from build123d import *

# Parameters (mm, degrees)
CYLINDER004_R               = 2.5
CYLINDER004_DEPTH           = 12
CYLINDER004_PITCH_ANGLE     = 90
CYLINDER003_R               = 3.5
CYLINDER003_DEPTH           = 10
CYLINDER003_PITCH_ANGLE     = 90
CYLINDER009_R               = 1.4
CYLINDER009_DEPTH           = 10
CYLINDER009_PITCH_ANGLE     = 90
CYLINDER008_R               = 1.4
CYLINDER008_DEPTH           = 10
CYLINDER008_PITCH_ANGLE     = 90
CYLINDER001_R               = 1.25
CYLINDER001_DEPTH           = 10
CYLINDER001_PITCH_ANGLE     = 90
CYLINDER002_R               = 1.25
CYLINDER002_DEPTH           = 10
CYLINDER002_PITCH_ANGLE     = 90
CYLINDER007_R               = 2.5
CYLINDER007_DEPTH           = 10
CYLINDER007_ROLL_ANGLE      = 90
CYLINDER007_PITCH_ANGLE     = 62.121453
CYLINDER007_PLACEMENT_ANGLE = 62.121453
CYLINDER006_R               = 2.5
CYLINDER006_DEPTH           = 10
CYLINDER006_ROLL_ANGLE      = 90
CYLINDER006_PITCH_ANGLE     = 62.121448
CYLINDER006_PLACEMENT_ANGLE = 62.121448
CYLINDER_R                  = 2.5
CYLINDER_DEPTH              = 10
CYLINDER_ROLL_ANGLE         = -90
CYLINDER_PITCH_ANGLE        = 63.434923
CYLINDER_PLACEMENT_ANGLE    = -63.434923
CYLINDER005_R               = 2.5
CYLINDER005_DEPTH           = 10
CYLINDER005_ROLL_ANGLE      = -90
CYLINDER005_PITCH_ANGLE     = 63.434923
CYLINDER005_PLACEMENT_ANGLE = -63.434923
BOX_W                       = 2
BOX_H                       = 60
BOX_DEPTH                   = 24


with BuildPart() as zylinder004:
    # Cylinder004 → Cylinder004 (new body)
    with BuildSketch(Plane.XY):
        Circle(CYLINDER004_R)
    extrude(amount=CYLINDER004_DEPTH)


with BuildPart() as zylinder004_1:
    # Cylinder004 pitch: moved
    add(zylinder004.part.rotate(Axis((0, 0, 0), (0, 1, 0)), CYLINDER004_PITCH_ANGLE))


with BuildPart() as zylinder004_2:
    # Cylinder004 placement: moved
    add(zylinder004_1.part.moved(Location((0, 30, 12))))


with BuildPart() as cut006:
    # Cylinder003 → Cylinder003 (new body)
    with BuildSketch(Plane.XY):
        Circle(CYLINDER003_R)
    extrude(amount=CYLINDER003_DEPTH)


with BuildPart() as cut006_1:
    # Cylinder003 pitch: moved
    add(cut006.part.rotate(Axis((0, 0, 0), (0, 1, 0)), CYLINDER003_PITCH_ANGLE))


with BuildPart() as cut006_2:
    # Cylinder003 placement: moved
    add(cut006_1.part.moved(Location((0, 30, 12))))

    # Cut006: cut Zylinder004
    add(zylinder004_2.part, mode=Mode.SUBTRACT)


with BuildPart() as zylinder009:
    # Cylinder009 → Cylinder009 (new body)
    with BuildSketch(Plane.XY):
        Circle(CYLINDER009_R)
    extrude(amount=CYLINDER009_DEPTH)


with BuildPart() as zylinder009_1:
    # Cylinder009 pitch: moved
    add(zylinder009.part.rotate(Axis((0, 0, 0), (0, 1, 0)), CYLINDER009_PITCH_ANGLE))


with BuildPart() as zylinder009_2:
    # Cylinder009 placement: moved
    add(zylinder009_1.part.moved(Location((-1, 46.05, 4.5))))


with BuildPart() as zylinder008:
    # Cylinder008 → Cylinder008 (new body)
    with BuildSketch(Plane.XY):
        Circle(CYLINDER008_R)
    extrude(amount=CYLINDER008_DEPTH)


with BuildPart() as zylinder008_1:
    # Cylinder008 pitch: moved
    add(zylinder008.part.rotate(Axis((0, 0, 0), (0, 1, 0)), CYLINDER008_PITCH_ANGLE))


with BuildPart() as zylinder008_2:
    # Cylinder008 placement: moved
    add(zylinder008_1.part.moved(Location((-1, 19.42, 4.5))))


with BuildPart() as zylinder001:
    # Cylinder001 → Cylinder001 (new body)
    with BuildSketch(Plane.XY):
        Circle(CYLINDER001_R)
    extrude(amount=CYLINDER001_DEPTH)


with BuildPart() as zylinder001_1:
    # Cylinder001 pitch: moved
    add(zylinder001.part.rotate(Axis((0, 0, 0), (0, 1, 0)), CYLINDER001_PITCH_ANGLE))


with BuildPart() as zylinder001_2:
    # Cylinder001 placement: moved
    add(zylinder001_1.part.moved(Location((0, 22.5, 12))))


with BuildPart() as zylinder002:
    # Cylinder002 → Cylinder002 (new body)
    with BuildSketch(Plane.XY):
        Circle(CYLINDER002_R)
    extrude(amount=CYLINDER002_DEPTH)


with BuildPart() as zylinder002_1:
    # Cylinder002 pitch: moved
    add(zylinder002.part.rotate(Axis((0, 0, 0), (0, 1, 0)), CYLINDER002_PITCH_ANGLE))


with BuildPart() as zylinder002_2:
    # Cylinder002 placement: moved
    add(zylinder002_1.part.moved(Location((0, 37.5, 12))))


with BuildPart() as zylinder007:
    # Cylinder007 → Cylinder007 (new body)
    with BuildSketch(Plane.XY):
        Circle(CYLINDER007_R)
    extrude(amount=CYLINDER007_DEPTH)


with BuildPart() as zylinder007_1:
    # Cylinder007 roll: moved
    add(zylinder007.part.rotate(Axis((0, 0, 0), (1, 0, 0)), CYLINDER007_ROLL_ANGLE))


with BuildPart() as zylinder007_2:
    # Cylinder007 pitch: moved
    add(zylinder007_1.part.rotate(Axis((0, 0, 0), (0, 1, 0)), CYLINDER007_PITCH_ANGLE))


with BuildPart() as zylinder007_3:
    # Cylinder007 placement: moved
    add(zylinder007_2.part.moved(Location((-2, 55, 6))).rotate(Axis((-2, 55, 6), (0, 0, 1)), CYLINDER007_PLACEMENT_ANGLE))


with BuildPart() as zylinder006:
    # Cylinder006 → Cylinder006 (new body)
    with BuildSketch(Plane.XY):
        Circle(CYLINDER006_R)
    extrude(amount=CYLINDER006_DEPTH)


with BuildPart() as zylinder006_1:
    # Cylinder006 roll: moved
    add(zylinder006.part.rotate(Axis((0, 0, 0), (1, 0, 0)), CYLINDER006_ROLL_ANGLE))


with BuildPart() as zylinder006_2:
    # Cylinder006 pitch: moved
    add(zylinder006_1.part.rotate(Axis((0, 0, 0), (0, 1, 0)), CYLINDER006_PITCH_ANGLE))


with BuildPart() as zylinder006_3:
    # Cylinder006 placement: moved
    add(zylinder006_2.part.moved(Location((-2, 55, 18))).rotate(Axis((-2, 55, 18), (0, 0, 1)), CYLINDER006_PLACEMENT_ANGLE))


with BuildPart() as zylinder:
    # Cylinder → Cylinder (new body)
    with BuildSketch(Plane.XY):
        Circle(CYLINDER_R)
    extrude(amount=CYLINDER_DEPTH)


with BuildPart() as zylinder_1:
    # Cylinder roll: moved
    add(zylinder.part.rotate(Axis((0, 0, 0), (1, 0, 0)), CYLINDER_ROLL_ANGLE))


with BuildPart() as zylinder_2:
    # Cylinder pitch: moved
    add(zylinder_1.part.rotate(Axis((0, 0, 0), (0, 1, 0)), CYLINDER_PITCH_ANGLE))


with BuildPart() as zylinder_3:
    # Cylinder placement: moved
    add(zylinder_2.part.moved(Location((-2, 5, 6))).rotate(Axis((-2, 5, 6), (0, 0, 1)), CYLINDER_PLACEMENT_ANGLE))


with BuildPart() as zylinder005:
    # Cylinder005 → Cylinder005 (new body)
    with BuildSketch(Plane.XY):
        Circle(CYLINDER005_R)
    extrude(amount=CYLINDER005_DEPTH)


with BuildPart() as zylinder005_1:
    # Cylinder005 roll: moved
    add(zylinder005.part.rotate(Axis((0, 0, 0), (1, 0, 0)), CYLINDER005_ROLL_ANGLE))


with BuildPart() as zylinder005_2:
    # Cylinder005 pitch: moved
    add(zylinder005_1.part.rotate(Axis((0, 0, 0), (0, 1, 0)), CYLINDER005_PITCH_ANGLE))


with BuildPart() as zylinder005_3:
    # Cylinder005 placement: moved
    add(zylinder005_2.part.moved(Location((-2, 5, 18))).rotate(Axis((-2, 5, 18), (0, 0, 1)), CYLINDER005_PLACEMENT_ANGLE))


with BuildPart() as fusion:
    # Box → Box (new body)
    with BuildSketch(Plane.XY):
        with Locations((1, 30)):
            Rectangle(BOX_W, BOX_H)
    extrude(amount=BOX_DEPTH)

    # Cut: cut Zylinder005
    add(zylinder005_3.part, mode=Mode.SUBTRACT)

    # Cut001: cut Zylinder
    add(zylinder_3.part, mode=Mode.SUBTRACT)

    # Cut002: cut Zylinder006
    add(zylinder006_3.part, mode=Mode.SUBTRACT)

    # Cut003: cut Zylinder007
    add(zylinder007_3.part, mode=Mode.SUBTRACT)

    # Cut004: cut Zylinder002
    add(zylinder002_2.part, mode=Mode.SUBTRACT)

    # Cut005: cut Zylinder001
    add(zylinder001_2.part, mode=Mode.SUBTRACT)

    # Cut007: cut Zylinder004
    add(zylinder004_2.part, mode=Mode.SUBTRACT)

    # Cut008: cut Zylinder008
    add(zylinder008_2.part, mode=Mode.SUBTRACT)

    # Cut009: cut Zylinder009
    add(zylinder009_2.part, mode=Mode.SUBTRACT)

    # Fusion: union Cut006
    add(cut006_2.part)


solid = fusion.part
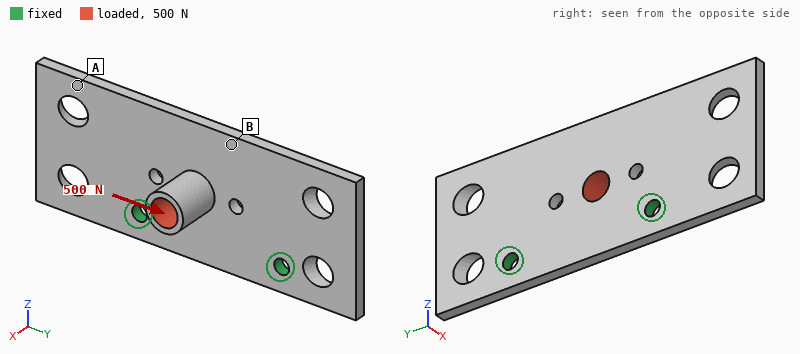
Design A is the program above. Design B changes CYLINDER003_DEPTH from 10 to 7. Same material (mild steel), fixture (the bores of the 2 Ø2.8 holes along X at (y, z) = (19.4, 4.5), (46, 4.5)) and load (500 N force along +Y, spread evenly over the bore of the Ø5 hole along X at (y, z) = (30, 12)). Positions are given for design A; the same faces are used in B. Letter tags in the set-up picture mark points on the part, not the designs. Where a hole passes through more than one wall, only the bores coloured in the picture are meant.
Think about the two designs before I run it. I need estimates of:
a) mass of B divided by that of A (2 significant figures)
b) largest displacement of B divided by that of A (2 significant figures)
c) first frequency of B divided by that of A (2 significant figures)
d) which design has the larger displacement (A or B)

0.98
0.48
1.0
A
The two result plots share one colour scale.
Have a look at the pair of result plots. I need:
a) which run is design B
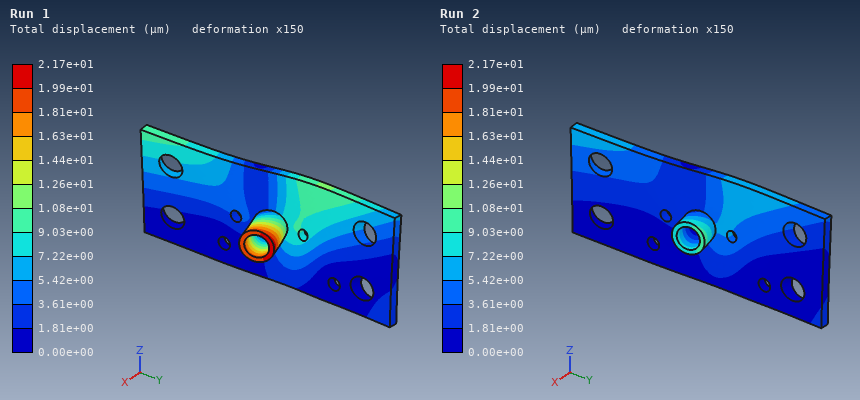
Run 2
